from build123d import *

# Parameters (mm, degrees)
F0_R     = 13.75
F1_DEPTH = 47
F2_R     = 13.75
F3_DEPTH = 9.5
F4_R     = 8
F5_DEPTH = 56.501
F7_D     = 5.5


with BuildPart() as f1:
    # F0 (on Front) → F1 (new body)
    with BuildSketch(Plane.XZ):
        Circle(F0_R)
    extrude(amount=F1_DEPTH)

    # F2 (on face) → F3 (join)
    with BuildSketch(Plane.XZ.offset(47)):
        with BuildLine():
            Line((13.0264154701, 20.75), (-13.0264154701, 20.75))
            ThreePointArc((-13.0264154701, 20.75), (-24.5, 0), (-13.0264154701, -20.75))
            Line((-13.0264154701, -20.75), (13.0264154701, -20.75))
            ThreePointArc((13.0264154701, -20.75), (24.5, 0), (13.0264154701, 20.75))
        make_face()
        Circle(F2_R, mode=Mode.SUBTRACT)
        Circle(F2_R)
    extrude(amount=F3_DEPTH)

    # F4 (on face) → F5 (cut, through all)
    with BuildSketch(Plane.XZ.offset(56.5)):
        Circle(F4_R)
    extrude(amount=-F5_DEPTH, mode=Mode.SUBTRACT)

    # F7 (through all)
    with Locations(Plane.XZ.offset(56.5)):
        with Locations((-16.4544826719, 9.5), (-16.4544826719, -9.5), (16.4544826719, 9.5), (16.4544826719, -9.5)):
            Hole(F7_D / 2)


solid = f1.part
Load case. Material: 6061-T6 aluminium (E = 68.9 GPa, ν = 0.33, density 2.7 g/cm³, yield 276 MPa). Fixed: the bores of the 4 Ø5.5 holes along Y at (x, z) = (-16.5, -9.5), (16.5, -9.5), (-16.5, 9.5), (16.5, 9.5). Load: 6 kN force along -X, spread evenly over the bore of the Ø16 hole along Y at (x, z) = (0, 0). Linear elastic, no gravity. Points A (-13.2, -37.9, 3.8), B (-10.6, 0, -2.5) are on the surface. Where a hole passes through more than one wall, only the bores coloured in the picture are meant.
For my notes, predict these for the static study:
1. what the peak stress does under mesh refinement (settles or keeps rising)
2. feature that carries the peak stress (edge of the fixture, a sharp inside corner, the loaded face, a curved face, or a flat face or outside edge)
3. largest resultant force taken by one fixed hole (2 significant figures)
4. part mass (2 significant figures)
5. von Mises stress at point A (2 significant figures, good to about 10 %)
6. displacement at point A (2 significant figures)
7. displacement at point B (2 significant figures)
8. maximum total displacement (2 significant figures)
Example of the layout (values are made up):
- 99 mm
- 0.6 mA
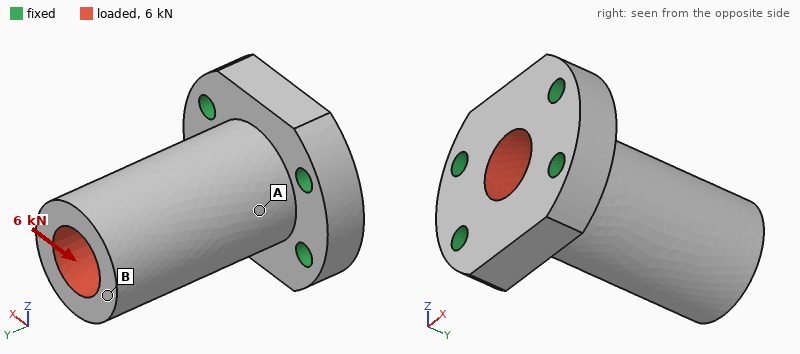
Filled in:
- keeps rising
- a sharp inside corner
- 3.0 kN
- 87 g
- 38 MPa
- 22 µm
- 84 µm
- 86 µm
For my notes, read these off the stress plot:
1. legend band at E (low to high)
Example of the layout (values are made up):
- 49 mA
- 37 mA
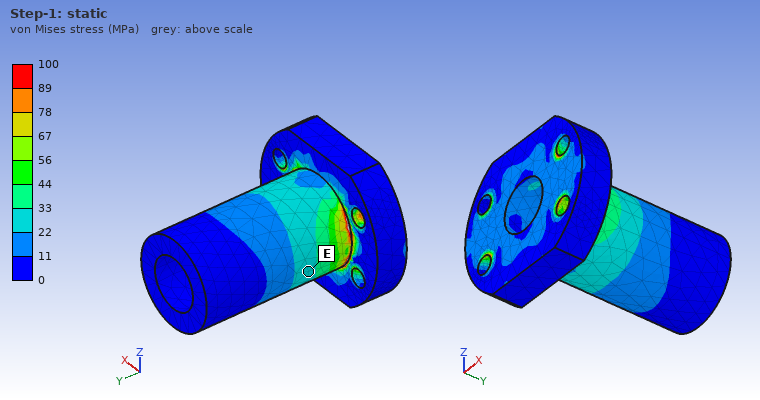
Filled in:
- 22 to 33 MPa
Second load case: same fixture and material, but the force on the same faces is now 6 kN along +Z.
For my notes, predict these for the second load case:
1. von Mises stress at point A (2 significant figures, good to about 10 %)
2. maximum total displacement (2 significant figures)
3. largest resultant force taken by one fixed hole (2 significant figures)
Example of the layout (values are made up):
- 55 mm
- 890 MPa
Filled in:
- 26 MPa
- 0.12 mm
- 3.4 kN
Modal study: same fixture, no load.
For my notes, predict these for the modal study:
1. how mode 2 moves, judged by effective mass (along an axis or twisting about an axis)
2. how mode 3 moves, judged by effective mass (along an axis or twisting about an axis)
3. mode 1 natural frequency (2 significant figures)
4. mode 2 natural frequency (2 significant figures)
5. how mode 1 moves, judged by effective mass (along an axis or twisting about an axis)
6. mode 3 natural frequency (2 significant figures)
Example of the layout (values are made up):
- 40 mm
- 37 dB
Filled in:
- along X
- twisting about Y
- 5600 Hz
- 6500 Hz
- along Z
- 15 kHz
